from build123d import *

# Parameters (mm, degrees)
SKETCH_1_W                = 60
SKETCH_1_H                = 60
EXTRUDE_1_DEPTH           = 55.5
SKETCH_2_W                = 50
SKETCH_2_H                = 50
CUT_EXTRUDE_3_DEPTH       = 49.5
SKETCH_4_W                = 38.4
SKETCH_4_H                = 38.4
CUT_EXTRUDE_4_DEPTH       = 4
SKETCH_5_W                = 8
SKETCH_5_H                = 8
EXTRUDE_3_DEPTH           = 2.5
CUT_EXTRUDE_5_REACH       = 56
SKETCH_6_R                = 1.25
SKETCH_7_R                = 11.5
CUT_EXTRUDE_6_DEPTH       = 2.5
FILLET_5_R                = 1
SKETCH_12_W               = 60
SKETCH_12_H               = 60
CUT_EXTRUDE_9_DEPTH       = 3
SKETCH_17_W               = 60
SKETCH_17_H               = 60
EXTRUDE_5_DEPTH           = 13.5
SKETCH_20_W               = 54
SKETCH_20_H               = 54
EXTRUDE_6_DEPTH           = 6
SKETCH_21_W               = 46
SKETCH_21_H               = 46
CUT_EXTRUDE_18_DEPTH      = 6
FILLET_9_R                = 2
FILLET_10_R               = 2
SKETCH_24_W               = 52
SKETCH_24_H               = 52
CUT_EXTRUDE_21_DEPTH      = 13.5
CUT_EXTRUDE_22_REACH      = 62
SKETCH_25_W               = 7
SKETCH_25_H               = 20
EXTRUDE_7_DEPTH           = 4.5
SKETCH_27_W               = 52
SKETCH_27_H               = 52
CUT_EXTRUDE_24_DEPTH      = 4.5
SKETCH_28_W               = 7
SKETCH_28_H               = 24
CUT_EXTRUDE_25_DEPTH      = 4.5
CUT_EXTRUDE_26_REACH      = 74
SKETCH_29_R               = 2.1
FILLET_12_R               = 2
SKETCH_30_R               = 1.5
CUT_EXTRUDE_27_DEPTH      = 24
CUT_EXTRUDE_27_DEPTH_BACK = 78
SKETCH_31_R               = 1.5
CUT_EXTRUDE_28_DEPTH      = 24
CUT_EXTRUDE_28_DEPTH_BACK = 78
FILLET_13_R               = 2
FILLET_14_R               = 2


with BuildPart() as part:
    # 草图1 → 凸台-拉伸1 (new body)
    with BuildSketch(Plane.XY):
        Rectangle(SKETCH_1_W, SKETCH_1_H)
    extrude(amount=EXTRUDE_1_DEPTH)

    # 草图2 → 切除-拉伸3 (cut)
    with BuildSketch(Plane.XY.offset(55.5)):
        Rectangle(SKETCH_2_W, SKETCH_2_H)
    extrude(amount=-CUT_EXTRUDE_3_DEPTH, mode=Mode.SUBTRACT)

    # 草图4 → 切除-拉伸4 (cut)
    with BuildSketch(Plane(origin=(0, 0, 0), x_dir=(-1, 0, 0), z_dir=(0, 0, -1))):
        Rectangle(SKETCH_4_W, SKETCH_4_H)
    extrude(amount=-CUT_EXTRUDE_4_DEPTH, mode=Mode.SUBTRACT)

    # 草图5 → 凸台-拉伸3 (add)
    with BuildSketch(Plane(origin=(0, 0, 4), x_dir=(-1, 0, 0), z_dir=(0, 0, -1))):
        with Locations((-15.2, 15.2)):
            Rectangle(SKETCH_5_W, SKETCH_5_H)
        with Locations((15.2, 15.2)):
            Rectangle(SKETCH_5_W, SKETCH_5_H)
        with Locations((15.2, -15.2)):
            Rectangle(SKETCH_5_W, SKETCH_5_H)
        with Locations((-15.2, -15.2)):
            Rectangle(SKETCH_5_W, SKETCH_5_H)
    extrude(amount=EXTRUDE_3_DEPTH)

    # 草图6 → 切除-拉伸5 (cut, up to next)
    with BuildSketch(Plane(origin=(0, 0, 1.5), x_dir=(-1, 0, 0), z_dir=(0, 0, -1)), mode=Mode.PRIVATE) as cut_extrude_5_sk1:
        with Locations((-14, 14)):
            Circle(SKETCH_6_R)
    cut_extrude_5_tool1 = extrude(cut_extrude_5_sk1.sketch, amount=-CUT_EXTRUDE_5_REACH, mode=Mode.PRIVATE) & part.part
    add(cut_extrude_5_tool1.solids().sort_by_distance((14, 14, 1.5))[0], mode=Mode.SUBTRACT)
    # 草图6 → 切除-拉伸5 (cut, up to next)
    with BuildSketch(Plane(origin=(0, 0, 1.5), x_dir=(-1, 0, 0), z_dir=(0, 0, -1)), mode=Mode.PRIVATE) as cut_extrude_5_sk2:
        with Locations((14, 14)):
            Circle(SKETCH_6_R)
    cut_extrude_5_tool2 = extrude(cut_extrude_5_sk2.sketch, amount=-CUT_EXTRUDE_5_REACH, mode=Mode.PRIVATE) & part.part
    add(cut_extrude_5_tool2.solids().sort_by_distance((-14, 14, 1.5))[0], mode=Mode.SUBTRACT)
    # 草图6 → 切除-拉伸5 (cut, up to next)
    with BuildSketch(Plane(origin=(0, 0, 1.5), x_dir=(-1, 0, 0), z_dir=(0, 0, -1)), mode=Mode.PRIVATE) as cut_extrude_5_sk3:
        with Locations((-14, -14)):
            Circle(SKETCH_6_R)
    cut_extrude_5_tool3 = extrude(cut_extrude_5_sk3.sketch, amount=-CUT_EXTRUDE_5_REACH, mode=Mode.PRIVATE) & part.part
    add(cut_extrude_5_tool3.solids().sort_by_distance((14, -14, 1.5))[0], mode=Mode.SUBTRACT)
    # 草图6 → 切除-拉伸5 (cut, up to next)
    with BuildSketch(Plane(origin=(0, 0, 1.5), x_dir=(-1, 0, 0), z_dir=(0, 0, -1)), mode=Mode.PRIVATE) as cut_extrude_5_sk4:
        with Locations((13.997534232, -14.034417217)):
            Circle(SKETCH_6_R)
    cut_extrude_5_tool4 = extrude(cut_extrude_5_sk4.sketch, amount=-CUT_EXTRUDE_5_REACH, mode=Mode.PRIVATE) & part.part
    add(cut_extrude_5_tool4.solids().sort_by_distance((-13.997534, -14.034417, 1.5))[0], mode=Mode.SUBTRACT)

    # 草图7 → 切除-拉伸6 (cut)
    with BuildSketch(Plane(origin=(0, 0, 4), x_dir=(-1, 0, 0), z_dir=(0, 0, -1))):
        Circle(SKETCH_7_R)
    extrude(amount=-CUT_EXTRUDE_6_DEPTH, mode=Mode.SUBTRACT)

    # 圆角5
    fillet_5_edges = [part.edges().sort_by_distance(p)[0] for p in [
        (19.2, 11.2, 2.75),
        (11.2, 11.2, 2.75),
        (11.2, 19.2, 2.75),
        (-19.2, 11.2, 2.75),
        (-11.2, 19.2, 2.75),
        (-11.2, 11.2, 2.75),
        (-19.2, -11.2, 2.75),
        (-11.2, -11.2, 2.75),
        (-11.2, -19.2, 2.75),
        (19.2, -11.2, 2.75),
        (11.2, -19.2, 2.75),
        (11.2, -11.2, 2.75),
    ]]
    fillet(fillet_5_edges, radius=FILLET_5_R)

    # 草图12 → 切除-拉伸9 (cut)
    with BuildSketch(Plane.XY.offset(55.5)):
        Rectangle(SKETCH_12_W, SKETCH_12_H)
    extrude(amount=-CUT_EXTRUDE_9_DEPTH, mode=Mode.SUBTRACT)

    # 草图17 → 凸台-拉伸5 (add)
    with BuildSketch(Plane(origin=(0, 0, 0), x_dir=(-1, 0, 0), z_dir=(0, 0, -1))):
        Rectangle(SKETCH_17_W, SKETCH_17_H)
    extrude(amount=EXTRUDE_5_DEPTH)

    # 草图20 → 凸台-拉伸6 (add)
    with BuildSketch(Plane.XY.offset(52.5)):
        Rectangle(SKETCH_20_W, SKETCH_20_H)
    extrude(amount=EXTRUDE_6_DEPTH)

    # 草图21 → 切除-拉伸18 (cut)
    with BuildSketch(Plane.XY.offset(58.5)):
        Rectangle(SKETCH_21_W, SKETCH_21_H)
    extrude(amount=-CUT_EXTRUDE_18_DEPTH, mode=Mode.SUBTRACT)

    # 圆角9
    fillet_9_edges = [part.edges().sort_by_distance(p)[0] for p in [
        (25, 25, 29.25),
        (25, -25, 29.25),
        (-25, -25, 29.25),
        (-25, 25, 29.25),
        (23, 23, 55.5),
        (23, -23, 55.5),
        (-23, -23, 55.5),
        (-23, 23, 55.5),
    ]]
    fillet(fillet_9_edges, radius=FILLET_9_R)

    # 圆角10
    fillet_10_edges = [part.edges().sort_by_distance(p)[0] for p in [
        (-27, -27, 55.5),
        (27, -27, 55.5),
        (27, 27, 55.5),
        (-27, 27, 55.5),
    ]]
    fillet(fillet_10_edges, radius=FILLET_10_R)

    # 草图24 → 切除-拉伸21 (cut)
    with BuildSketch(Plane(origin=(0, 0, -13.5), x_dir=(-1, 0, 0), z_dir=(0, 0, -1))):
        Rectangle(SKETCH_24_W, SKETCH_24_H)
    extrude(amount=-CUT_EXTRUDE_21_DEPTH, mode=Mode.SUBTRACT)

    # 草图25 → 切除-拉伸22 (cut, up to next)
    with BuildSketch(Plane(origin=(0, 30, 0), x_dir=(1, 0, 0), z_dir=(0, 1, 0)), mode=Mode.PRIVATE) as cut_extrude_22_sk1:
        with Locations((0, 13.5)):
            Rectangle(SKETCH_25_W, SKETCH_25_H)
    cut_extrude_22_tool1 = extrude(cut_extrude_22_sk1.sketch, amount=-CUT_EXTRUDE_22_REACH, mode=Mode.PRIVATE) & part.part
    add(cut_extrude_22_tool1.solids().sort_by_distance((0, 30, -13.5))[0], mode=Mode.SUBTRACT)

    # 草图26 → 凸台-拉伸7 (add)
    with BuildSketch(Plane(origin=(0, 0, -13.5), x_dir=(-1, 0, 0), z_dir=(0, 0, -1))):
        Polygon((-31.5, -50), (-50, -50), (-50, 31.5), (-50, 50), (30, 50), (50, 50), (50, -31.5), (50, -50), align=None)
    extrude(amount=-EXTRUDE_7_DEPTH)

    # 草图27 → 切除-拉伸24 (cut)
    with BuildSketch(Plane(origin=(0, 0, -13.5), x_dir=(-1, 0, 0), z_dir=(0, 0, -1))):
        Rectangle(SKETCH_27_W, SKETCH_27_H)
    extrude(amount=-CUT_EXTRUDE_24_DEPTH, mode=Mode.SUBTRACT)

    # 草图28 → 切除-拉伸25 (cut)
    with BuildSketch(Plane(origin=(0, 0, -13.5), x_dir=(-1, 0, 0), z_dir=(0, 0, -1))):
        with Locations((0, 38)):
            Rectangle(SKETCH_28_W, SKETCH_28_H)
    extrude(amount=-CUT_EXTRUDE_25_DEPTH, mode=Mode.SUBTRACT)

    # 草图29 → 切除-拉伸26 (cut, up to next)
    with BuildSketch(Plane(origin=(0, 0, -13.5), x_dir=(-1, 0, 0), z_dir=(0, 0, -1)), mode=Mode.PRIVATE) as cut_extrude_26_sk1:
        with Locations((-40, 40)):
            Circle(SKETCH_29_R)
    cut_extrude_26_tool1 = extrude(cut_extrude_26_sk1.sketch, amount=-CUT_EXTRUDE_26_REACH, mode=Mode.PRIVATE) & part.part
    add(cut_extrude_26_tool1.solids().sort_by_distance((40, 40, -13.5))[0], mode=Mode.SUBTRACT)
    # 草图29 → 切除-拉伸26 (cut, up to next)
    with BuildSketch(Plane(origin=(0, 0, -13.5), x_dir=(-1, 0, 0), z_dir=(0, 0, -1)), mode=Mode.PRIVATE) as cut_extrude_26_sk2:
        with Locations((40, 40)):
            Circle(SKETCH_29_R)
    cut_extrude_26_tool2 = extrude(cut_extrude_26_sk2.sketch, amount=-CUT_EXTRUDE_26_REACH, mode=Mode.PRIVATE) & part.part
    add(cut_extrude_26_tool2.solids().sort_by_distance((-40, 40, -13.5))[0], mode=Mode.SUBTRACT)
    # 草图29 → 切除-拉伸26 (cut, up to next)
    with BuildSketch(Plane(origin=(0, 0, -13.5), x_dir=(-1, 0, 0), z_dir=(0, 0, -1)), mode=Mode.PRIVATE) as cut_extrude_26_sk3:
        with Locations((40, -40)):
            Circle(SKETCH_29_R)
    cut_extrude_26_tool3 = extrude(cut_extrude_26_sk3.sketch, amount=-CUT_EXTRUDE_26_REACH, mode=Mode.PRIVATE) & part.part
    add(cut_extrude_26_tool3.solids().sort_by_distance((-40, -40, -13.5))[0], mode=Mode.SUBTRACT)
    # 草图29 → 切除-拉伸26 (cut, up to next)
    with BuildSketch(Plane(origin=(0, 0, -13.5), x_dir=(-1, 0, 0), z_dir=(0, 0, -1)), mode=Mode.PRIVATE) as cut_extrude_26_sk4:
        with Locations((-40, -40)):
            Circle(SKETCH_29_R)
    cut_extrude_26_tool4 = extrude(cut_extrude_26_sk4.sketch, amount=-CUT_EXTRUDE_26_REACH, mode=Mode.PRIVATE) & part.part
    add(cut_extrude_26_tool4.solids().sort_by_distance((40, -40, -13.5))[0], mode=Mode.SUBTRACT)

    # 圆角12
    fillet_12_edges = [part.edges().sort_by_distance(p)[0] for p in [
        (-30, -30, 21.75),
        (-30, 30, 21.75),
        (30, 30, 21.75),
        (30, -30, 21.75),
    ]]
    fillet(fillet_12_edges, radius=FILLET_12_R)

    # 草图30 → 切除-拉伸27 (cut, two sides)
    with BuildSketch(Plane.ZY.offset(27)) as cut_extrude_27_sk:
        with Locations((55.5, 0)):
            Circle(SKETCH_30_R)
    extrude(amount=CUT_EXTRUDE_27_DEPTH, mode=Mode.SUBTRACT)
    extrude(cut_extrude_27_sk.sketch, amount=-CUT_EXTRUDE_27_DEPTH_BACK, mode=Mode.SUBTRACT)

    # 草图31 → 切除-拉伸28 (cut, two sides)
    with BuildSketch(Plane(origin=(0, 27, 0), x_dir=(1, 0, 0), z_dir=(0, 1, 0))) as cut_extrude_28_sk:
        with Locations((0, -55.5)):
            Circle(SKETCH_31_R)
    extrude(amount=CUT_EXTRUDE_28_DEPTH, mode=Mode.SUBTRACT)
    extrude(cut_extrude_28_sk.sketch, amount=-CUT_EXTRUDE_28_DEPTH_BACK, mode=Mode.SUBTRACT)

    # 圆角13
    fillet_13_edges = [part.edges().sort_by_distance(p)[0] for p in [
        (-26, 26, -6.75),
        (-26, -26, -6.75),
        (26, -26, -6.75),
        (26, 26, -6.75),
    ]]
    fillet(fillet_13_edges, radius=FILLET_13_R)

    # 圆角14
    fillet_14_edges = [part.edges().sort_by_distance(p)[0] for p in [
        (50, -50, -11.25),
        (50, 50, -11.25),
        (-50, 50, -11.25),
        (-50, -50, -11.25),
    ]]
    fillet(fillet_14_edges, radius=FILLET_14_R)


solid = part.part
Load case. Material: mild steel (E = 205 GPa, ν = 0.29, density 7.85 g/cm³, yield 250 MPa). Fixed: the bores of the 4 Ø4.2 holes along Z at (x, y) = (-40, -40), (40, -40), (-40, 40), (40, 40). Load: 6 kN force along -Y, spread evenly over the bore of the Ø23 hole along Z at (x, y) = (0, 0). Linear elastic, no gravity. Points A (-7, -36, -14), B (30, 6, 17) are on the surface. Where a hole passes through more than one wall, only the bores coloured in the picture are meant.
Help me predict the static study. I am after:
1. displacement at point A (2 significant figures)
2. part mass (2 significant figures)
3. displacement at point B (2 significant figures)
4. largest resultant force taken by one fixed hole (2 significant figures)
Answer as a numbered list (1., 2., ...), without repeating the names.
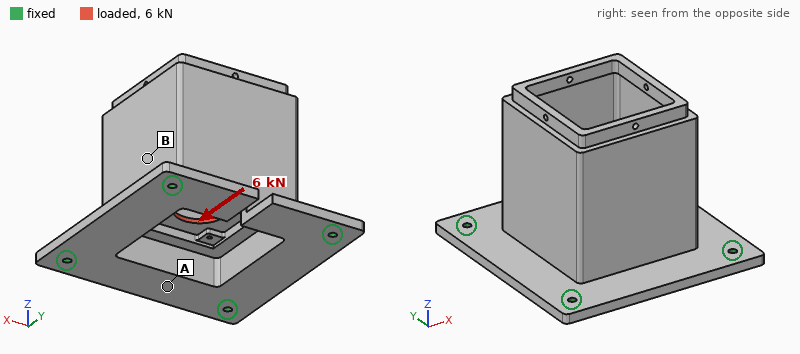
1. 13 µm
2. 870 g
3. 15 µm
4. 1.8 kN
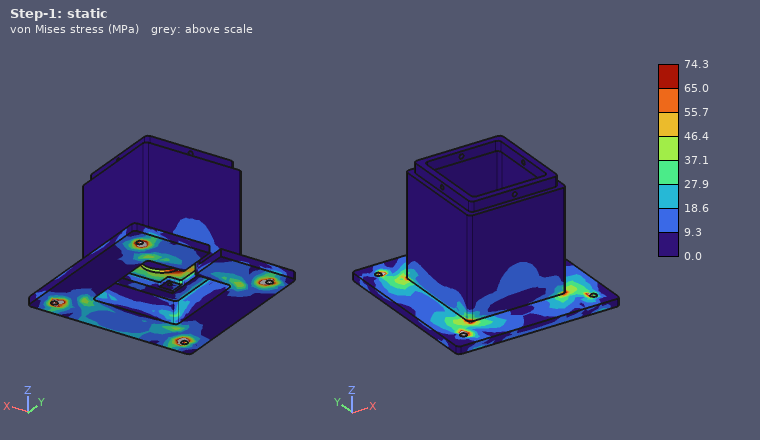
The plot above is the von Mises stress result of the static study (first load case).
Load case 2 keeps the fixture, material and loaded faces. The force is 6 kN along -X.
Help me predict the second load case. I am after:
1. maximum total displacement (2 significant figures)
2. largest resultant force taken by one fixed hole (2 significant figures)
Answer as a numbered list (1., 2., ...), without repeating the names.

1. 31 µm
2. 1.9 kN
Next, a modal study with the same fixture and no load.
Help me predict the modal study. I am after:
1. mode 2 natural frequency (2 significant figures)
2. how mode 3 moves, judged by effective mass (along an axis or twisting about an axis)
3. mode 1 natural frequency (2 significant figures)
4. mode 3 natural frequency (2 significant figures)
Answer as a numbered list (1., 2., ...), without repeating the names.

1. 2000 Hz
2. along Z
3. 2000 Hz
4. 2500 Hz
